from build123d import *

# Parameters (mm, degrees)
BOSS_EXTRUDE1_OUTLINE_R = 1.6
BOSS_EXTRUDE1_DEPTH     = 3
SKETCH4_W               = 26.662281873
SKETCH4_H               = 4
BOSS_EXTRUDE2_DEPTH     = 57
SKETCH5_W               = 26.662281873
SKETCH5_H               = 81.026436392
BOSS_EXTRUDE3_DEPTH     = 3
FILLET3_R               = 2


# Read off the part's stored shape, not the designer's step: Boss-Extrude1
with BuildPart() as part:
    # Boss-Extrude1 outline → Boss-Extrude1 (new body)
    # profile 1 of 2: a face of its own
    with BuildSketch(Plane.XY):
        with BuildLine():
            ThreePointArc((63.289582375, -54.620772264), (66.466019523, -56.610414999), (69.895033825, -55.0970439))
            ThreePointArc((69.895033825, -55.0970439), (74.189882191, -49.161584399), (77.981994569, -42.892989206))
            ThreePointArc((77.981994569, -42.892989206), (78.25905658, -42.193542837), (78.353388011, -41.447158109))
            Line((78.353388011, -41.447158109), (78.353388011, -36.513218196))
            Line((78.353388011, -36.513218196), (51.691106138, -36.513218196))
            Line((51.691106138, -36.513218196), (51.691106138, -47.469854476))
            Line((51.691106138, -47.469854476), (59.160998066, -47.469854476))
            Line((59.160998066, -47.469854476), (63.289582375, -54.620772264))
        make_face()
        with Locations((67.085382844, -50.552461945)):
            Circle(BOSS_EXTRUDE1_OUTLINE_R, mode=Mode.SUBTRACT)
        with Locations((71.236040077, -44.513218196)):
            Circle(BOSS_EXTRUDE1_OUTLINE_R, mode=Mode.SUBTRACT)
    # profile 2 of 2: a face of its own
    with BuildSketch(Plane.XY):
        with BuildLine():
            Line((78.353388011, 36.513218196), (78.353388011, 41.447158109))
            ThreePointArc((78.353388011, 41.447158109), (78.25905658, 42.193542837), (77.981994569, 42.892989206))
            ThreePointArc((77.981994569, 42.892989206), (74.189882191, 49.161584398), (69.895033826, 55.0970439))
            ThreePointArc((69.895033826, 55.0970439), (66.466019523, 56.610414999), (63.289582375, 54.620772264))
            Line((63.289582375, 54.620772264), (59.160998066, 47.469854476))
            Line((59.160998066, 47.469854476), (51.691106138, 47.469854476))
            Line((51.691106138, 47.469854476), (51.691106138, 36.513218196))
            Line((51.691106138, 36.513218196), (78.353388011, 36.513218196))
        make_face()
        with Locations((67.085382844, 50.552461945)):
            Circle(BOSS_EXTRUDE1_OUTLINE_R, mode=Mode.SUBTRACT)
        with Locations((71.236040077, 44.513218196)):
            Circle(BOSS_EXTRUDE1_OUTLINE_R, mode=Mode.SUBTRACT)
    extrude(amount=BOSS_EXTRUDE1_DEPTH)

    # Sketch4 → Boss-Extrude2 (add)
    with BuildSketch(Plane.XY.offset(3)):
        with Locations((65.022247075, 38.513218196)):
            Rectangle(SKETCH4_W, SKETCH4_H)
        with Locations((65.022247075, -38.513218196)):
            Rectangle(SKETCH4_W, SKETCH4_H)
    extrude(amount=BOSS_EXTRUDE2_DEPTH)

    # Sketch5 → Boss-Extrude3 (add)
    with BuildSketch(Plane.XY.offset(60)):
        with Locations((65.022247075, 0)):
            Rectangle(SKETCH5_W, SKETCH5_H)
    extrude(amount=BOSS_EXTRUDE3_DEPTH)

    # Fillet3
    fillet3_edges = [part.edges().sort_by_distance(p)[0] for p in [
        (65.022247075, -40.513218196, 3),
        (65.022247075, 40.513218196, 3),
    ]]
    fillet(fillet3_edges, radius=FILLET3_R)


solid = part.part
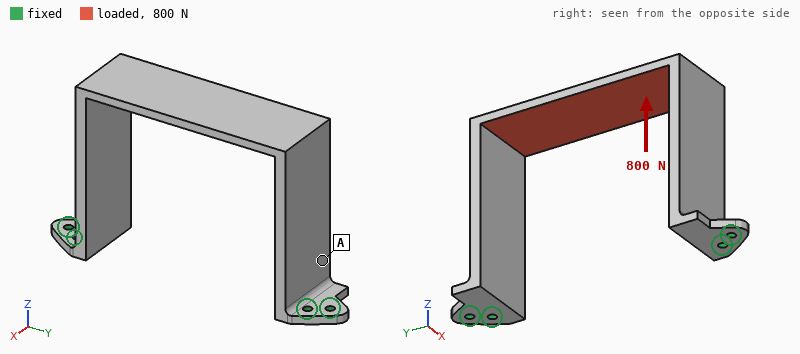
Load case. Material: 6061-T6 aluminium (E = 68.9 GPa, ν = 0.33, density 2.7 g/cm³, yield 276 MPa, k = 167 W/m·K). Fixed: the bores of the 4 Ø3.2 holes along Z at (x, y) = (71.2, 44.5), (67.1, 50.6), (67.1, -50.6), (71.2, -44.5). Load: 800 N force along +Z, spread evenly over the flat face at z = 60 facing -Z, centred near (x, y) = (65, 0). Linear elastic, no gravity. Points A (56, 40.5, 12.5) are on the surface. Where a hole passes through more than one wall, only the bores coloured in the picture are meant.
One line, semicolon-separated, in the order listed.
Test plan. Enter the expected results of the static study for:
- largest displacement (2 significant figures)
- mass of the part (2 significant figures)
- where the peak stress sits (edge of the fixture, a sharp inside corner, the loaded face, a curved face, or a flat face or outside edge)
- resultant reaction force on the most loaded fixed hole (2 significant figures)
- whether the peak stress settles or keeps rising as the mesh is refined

0.39 mm; 56 g; edge of the fixture; 250 N; keeps rising
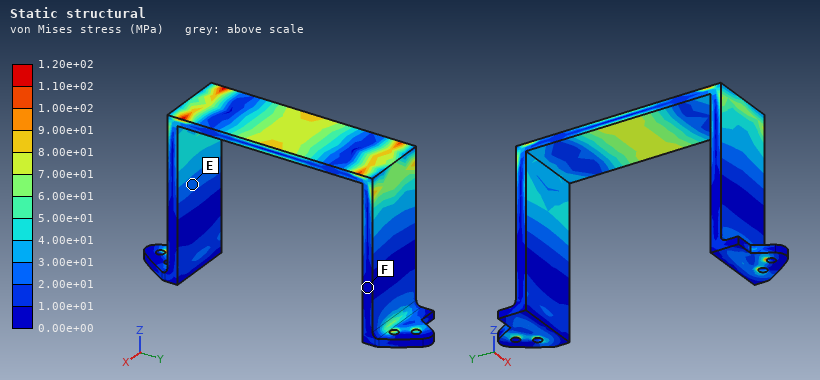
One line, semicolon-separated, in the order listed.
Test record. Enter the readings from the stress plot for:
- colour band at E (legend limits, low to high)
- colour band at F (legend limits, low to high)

2.00e+01 to 3.00e+01 MPa; 0.00e+00 to 1.00e+01 MPa
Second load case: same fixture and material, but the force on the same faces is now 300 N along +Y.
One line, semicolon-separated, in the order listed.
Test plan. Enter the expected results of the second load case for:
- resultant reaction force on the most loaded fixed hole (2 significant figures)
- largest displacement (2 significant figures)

310 N; 0.75 mm
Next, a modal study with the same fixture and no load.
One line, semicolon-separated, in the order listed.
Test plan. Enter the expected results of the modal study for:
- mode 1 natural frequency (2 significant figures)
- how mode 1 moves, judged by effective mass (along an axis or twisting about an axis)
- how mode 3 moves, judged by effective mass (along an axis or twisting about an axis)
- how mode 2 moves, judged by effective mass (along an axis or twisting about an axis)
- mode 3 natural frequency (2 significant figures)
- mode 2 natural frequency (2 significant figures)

610 Hz; along Y; twisting about Z; along X; 1200 Hz; 770 Hz
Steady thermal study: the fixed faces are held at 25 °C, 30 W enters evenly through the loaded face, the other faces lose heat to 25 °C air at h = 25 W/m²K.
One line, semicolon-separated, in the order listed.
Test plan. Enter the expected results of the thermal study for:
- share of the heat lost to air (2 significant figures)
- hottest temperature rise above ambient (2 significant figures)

29 %; 64 K
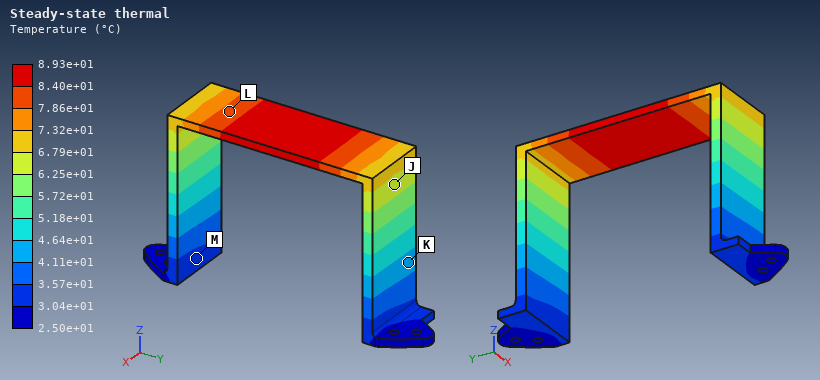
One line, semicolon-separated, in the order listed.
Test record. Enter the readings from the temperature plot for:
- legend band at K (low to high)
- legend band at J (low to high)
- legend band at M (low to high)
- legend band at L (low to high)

4.11e+01 to 4.64e+01 °C; 6.25e+01 to 6.79e+01 °C; 3.04e+01 to 3.57e+01 °C; 7.86e+01 to 8.40e+01 °C
